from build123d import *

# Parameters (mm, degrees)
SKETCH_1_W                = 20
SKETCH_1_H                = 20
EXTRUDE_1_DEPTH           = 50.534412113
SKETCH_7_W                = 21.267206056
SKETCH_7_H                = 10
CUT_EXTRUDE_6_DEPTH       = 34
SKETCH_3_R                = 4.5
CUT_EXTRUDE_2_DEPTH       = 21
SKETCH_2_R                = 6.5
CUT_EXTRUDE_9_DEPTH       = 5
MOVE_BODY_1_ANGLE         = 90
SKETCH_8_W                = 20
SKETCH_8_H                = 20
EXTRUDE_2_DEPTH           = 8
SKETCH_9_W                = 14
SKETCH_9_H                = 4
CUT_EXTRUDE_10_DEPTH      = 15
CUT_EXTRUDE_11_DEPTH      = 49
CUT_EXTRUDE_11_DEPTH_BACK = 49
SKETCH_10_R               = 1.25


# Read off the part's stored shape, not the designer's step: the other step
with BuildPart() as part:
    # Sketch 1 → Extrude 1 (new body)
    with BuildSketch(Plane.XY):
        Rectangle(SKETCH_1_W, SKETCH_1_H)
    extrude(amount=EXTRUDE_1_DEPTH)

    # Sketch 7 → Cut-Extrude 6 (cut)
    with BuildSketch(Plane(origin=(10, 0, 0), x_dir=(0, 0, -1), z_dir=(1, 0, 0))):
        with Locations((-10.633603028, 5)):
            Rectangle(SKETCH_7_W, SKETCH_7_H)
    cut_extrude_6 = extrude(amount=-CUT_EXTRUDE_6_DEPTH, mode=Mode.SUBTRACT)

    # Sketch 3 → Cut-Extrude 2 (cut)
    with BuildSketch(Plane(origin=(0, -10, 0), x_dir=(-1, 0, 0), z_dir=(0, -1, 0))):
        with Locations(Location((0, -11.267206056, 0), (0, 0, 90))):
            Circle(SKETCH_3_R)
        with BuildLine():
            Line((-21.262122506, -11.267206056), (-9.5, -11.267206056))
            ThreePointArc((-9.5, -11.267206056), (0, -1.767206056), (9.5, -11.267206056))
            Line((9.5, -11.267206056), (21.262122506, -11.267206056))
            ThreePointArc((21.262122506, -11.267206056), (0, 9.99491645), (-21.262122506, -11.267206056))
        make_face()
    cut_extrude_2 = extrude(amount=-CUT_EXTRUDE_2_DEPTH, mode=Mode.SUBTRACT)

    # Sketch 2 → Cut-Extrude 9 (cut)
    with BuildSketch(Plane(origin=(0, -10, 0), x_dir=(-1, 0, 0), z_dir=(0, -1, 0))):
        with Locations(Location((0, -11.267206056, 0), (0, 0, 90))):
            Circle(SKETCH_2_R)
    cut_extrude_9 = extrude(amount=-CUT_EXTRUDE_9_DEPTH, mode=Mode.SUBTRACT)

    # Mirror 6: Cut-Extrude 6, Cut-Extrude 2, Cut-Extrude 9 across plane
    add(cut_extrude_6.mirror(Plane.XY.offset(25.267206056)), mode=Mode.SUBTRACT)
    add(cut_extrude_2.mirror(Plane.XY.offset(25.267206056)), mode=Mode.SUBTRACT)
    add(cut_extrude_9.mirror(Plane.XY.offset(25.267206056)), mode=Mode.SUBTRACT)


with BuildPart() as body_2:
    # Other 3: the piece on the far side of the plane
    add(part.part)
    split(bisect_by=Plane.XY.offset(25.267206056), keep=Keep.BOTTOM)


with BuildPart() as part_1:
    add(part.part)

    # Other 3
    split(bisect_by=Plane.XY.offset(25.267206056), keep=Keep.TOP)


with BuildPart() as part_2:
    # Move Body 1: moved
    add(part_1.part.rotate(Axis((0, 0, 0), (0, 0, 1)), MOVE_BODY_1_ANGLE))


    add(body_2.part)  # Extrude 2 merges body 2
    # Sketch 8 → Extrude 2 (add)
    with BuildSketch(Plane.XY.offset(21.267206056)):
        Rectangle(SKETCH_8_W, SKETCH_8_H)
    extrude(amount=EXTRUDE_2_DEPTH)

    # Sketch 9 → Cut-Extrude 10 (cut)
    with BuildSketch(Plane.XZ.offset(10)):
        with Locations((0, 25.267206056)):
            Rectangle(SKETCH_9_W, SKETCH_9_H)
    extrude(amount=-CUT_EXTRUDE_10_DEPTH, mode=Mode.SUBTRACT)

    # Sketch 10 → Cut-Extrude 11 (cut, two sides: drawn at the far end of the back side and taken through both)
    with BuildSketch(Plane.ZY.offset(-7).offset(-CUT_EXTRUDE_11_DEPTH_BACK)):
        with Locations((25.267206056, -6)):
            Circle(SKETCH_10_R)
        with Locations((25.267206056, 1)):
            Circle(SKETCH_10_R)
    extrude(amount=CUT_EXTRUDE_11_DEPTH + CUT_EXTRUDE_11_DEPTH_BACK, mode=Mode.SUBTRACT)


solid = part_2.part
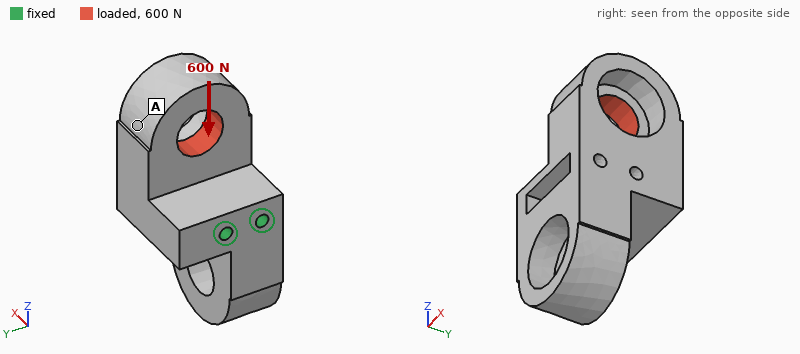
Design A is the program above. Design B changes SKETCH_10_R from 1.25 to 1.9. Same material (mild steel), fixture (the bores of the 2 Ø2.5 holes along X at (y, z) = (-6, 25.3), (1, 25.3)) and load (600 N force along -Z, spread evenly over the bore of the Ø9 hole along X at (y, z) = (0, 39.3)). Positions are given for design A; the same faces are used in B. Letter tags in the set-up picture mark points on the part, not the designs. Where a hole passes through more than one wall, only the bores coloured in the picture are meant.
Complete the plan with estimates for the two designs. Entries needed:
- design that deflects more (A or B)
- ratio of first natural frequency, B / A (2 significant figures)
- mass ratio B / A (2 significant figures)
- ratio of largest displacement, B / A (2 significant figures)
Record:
A
1.2
0.99
0.68
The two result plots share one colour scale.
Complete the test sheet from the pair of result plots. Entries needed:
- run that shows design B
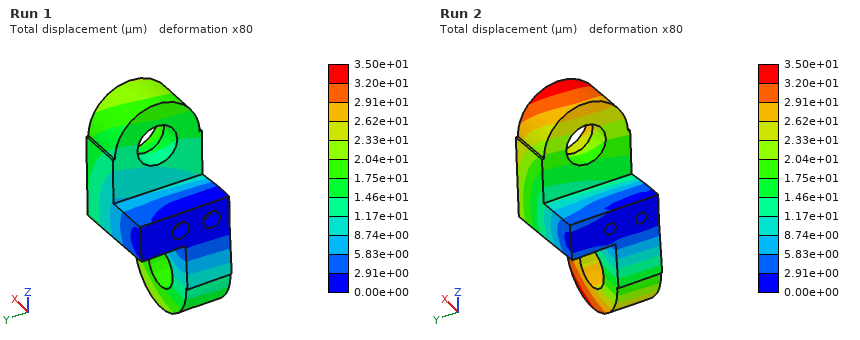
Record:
Run 1
